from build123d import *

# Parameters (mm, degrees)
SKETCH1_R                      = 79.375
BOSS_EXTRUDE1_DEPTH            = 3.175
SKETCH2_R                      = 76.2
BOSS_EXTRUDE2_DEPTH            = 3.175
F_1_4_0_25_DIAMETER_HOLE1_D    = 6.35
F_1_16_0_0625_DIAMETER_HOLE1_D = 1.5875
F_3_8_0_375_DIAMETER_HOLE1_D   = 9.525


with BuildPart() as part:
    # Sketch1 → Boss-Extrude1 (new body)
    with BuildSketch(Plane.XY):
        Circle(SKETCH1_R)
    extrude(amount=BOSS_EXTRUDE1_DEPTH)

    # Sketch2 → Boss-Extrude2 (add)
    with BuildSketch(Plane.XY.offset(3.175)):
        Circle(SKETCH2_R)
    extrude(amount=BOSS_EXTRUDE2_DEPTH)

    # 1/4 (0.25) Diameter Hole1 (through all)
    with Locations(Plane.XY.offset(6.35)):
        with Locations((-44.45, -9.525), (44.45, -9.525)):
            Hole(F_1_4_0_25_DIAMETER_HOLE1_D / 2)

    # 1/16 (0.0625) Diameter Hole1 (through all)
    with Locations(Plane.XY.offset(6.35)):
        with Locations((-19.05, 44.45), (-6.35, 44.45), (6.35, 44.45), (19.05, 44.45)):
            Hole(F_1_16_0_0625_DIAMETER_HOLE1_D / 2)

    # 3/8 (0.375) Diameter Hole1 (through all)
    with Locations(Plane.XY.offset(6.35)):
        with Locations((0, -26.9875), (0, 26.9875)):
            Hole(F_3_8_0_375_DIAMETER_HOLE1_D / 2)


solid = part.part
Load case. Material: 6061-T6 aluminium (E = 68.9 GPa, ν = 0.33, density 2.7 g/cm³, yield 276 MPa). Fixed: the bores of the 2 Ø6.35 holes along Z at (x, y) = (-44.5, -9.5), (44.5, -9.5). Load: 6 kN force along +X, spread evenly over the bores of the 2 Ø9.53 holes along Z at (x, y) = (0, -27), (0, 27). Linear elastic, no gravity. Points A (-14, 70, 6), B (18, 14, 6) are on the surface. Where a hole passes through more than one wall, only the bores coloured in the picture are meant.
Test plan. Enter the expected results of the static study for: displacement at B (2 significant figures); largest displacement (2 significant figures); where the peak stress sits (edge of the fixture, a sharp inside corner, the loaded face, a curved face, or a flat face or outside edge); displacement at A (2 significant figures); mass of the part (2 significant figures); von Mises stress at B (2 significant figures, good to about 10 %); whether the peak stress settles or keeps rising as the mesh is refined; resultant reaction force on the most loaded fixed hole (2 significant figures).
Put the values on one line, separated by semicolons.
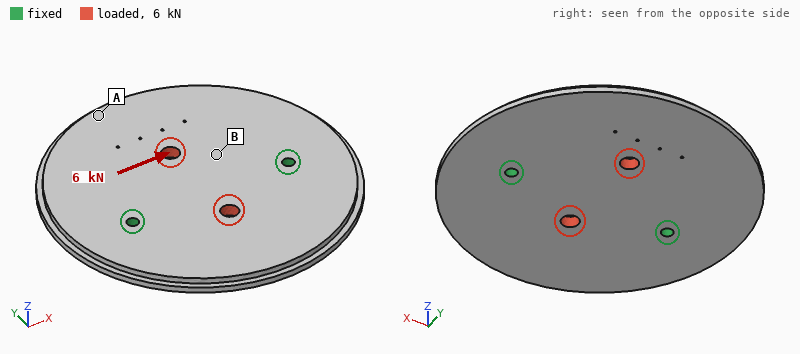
6.8 µm; 12 µm; edge of the fixture; 9.6 µm; 320 g; 8.7 MPa; keeps rising; 3.1 kN
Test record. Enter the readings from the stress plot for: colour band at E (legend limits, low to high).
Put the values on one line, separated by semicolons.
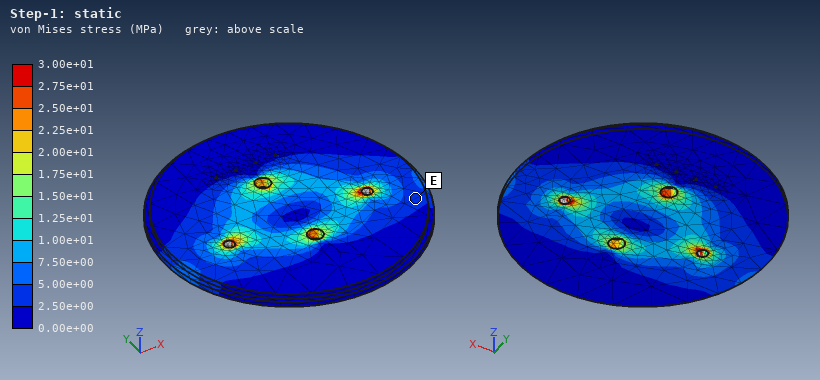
2.50e+00 to 5.00e+00 MPa
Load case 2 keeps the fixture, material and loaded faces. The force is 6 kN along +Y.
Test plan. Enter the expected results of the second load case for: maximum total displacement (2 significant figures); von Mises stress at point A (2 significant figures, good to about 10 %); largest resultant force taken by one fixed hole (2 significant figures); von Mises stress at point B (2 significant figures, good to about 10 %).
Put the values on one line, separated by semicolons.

12 µm; 4.1 MPa; 3.0 kN; 8.1 MPa
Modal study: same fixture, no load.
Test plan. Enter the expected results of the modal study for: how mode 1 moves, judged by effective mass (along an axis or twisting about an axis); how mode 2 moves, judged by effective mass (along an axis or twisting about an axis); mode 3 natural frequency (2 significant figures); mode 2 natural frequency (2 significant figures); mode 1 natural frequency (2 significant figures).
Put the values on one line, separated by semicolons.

along Z; along Z; 1700 Hz; 1200 Hz; 740 Hz
